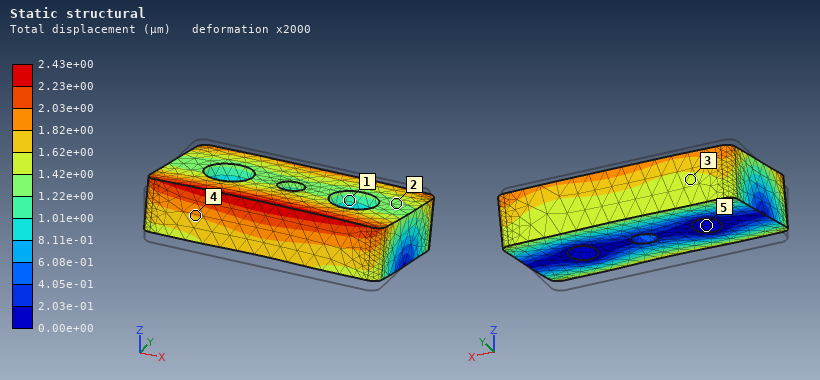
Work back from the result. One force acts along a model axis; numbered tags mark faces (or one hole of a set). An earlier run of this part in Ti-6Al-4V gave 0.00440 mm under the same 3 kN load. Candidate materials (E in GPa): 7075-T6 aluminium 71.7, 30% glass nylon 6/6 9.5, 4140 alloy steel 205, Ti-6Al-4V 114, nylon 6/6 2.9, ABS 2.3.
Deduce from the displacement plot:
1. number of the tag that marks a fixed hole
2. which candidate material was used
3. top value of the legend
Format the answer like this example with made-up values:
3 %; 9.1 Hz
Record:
5; 4140 alloy steel; 2.43e+00 µm
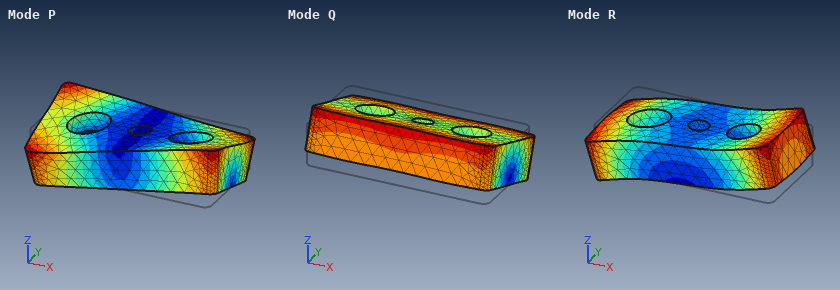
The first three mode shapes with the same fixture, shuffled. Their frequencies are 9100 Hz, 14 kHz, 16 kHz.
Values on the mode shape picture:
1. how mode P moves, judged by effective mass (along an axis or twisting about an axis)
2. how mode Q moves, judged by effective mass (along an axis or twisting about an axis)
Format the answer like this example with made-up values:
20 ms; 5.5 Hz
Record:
twisting about Z; along Y
